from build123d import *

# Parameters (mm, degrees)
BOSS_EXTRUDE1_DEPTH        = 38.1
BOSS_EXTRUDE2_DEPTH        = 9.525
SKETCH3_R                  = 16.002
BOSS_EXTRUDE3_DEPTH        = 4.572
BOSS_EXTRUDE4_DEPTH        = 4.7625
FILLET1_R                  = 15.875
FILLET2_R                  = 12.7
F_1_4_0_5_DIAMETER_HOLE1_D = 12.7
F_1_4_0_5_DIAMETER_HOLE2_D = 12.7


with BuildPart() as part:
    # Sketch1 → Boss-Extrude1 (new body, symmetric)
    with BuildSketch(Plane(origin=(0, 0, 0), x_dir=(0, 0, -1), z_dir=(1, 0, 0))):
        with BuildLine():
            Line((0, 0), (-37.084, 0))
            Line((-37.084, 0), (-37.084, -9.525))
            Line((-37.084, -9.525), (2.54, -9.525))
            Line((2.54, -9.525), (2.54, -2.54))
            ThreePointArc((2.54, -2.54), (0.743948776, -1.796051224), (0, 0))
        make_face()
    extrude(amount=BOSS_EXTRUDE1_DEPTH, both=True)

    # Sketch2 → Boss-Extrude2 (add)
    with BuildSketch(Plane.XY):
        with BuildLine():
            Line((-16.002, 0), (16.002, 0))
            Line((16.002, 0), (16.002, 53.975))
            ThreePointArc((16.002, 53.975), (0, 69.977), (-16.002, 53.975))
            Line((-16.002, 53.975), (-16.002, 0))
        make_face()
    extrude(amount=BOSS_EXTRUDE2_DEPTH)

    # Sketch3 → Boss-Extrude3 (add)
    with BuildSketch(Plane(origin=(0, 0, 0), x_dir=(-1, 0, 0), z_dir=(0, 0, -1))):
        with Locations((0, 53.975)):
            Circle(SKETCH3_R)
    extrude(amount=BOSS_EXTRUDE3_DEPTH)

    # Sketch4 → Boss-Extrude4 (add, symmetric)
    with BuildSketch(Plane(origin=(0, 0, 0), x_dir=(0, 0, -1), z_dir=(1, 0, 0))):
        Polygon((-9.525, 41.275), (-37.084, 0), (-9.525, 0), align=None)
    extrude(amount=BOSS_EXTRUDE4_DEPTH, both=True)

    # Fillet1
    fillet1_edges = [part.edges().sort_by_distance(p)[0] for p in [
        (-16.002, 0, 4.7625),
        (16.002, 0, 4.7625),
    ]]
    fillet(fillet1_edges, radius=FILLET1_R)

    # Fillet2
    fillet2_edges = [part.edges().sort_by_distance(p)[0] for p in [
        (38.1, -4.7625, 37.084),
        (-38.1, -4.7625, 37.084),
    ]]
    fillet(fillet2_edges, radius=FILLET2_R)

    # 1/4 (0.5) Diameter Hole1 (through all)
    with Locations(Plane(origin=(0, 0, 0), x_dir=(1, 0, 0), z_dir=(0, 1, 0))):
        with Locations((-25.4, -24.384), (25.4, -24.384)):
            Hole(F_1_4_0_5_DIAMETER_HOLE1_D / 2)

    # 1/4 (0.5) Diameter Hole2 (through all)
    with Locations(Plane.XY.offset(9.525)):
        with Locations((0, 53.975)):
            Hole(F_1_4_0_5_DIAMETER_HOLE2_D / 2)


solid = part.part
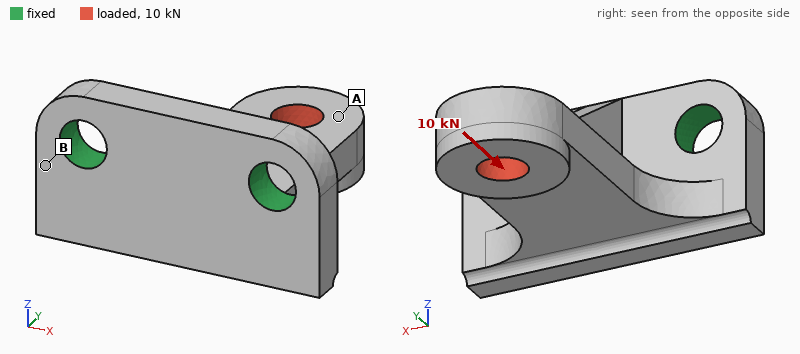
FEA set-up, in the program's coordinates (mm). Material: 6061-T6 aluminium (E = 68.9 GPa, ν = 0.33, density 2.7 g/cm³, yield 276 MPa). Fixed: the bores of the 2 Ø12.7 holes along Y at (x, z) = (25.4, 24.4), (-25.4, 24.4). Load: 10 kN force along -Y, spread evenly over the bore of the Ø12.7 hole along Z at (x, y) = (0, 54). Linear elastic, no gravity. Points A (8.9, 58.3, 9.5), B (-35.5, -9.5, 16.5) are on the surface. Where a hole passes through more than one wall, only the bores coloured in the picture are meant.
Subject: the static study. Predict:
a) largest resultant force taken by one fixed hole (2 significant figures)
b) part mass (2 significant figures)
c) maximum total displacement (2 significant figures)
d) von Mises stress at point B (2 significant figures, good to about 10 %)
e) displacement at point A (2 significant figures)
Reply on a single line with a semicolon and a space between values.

5.1 kN; 150 g; 0.42 mm; 80 MPa; 0.32 mm
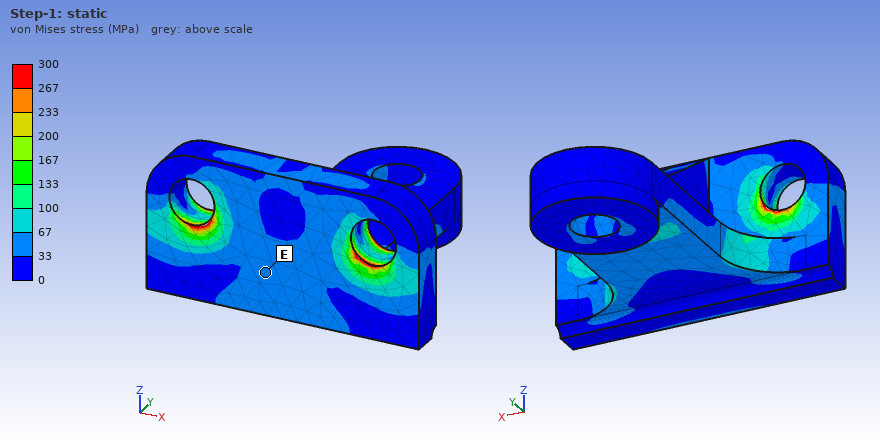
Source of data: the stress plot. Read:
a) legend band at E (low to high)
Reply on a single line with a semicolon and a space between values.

33 to 67 MPa
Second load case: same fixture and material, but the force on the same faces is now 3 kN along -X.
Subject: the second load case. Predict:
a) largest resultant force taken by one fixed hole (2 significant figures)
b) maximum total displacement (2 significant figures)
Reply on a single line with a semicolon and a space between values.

4.3 kN; 0.22 mm
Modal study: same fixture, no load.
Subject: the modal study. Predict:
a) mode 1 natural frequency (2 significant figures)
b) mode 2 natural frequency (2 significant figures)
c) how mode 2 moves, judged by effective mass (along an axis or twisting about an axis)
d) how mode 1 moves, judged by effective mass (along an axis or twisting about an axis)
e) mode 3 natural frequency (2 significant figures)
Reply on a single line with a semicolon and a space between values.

2300 Hz; 3700 Hz; along X; along Z; 7300 Hz
